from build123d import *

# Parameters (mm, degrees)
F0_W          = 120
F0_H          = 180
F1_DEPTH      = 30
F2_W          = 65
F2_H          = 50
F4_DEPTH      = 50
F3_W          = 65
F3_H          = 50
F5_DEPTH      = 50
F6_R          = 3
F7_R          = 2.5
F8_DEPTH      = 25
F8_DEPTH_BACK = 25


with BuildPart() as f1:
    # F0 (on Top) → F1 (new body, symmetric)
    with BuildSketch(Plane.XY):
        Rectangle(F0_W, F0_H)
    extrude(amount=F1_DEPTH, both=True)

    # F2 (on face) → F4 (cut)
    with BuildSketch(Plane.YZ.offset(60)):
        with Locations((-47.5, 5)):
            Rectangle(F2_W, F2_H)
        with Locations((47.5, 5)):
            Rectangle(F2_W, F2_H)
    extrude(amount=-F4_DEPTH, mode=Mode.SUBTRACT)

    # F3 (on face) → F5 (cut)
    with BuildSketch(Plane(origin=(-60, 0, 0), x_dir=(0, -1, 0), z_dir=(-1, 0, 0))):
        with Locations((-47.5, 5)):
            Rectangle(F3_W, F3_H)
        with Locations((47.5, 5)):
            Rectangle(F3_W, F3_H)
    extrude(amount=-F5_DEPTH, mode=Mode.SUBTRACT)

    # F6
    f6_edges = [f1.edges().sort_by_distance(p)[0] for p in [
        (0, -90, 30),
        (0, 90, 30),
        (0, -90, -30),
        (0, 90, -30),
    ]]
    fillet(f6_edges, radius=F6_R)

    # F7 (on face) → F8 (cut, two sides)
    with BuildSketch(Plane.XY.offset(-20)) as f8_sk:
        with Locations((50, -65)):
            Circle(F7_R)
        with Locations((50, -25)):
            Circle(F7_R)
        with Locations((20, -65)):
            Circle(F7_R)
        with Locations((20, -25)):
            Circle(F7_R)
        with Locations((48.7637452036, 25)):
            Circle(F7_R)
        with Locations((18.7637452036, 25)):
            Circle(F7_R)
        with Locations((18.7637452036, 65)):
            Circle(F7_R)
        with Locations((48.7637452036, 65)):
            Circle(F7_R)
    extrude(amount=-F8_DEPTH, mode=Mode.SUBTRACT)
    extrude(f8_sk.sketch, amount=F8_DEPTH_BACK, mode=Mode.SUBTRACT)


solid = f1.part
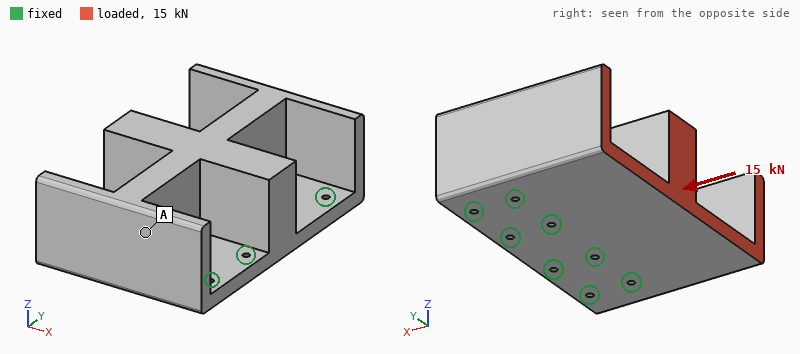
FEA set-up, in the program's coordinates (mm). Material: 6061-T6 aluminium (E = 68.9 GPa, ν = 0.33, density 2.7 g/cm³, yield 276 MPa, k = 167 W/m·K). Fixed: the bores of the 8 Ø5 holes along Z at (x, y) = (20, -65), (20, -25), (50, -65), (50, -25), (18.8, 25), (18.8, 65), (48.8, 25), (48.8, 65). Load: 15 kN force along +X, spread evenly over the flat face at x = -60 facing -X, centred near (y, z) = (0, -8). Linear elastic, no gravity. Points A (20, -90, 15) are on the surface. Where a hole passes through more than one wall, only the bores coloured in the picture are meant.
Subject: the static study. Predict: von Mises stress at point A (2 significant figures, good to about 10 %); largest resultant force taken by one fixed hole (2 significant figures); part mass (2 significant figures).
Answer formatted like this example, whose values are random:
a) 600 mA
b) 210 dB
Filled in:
a) 5.2 MPa
b) 3.2 kN
c) 1.7 kg
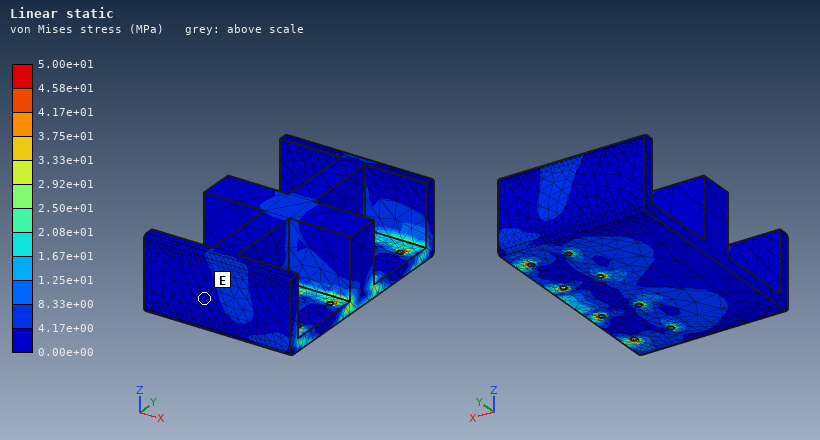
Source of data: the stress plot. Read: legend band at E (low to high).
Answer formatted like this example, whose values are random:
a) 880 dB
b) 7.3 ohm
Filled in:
a) 0.00e+00 to 4.17e+00 MPa
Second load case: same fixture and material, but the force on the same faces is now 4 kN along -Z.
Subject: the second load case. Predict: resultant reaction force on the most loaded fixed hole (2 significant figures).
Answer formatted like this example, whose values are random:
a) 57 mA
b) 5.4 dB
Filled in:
a) 3.5 kN
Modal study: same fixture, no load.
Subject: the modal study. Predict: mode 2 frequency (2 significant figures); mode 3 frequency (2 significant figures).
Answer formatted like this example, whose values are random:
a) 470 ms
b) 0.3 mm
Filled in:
a) 2300 Hz
b) 3800 Hz
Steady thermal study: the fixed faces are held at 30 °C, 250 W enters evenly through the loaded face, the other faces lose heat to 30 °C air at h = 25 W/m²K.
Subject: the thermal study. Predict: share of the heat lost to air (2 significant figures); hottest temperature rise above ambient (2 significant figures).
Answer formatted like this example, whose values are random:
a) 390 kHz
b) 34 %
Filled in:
a) 14 %
b) 34 K
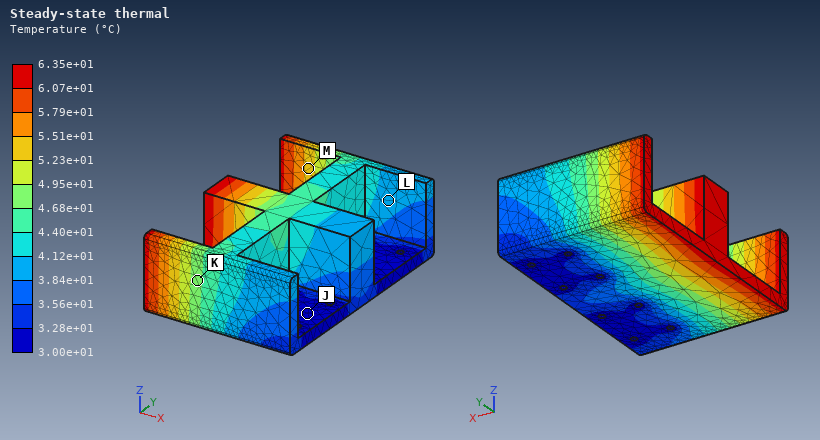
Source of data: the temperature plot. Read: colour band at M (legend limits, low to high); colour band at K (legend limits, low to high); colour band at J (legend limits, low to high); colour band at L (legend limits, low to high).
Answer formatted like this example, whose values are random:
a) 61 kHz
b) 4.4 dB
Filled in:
a) 5.23e+01 to 5.51e+01 °C
b) 4.68e+01 to 4.95e+01 °C
c) 3.00e+01 to 3.28e+01 °C
d) 3.84e+01 to 4.12e+01 °C
